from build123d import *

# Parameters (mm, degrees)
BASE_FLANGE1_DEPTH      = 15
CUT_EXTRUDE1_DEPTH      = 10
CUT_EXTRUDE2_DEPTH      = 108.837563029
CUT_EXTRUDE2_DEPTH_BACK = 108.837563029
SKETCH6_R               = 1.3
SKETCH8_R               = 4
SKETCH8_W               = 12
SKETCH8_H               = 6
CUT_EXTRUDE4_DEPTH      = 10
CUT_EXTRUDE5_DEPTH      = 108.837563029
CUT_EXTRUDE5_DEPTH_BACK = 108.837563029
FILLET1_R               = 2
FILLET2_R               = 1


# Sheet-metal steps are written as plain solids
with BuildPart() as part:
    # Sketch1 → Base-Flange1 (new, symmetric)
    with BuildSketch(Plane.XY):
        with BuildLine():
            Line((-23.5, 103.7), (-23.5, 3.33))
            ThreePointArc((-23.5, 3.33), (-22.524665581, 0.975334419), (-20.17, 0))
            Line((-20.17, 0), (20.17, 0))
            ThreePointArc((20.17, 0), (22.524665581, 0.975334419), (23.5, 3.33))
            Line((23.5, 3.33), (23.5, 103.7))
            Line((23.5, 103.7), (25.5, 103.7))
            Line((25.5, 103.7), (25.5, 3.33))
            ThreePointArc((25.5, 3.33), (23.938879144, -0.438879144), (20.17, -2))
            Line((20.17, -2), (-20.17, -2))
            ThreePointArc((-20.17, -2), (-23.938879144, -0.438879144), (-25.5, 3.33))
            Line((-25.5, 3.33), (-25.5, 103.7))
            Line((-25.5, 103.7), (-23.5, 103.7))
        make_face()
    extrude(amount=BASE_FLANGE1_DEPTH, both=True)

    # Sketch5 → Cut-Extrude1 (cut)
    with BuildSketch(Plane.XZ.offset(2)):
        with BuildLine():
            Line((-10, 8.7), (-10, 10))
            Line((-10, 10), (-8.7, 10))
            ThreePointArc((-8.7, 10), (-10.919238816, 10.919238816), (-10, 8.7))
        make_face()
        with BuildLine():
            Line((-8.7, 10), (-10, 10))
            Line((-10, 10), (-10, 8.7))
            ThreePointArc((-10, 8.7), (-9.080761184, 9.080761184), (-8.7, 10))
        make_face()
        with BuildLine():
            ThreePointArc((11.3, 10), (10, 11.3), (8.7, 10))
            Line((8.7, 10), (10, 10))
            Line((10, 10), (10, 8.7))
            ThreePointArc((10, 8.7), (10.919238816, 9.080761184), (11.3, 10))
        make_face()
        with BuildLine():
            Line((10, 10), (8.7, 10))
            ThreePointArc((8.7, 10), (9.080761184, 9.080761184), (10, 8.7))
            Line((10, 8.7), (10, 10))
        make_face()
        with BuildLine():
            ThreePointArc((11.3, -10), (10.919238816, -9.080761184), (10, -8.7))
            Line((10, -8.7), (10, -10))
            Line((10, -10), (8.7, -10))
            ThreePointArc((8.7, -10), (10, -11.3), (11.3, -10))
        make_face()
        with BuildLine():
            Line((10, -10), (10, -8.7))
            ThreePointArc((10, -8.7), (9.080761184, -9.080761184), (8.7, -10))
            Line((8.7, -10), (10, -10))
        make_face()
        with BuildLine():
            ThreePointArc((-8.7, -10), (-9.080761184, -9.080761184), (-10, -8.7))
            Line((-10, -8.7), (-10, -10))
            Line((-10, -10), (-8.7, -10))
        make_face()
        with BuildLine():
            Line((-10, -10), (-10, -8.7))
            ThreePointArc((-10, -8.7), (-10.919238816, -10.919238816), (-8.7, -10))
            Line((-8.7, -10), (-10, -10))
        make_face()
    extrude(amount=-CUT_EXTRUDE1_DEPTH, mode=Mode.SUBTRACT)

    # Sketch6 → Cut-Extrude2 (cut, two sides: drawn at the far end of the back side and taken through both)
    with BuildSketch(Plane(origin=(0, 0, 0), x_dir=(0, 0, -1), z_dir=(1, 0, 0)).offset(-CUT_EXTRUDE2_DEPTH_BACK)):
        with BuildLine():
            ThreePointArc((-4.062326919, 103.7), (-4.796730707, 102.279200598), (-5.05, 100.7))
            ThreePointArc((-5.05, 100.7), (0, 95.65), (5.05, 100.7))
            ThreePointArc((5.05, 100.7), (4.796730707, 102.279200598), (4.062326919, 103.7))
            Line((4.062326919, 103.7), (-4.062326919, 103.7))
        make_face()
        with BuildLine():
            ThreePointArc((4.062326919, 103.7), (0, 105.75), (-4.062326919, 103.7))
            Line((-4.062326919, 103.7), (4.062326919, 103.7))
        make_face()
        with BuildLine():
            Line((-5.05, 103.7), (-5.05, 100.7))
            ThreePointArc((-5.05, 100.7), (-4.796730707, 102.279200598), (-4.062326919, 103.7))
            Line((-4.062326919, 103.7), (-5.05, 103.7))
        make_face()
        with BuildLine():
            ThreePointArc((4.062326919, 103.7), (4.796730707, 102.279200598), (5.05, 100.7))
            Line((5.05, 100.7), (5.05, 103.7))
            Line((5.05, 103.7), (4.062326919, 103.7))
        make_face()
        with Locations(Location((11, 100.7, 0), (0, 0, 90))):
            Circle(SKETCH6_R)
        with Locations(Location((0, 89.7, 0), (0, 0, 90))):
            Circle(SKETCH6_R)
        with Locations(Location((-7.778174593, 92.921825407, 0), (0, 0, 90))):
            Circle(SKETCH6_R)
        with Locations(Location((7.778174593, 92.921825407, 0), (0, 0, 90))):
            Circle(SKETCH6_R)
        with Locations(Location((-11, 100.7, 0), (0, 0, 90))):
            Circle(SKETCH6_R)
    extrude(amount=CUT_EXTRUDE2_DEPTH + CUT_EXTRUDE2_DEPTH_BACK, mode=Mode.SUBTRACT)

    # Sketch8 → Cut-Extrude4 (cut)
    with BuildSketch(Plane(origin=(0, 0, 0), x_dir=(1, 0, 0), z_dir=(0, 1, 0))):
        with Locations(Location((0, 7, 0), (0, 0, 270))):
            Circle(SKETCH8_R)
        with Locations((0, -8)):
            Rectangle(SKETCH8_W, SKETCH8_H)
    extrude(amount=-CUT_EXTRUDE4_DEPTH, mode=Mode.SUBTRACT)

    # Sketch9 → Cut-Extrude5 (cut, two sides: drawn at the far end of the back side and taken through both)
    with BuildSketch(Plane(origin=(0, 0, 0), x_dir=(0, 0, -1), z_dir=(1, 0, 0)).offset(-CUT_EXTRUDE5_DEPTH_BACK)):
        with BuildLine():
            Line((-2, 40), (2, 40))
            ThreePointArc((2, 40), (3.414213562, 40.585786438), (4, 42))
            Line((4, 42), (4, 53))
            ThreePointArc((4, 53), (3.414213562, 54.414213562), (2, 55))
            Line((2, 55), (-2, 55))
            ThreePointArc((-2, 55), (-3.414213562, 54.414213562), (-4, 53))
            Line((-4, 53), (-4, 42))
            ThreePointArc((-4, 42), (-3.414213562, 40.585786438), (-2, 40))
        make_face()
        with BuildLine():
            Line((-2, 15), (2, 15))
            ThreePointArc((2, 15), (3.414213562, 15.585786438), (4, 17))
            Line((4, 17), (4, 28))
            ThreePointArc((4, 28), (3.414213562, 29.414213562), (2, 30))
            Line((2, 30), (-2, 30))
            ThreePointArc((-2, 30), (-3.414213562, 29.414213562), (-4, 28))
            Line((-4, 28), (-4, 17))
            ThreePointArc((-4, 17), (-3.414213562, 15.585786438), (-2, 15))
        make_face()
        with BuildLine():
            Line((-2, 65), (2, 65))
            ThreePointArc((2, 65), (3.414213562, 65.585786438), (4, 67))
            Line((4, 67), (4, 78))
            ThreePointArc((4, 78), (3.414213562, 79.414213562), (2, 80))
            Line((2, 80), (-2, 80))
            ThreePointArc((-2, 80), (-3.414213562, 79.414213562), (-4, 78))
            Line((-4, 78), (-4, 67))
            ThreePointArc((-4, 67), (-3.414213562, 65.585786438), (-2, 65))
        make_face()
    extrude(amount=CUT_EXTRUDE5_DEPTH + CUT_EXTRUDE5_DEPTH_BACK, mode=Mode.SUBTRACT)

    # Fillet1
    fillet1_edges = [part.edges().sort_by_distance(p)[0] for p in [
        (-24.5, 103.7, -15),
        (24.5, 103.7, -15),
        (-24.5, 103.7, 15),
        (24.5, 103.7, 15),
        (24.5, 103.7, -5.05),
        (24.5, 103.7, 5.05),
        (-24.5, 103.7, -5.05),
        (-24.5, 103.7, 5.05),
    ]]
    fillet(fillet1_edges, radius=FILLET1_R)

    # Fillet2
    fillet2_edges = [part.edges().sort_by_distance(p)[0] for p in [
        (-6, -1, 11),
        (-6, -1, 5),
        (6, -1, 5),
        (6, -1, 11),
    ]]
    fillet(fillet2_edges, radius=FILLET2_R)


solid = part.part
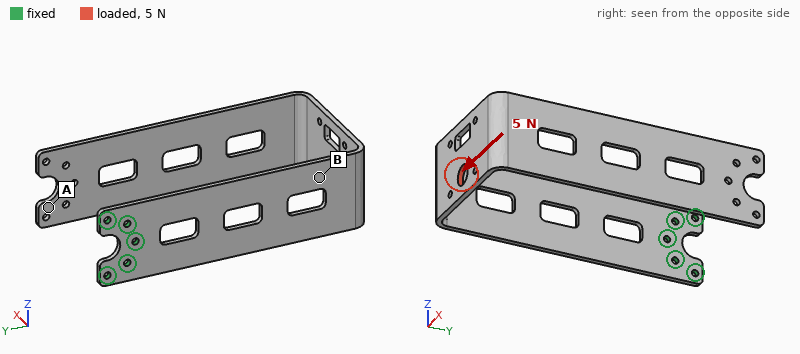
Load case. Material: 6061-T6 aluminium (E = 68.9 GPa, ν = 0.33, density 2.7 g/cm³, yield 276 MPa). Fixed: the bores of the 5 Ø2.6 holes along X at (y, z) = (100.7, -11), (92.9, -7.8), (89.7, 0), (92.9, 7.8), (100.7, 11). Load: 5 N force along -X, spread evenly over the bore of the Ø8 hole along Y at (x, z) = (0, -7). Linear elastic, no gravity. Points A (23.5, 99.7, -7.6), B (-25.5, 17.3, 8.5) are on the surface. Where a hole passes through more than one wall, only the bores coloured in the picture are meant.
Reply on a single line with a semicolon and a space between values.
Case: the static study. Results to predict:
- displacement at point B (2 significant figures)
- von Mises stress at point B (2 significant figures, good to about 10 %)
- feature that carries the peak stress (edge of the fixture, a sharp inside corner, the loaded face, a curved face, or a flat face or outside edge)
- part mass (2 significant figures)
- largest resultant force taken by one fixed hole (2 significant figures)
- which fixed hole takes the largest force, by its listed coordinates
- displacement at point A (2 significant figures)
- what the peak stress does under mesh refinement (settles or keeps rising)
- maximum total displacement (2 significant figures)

0.77 mm; 6.6 MPa; edge of the fixture; 36 g; 30 N; (89.7, 0); 1.2 mm; keeps rising; 1.4 mm
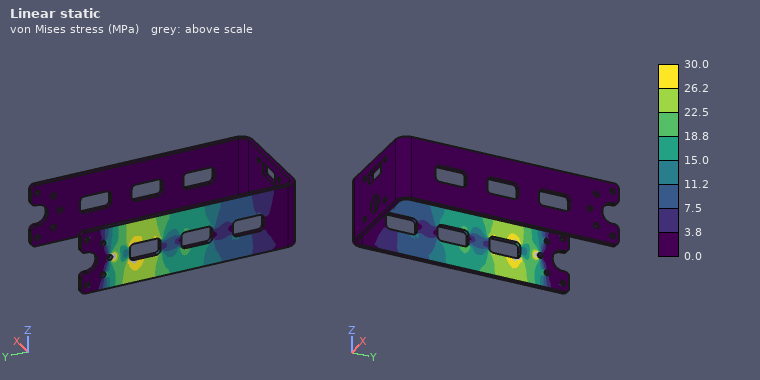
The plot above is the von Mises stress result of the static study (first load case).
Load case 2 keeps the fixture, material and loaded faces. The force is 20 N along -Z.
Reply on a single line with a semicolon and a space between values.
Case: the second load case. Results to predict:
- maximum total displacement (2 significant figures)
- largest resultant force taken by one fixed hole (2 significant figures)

1.4 mm; 67 N
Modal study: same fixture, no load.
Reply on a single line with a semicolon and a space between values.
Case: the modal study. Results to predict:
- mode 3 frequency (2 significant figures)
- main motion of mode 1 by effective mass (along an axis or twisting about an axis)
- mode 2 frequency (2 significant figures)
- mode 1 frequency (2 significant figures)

88 Hz; along Y; 87 Hz; 60 Hz
